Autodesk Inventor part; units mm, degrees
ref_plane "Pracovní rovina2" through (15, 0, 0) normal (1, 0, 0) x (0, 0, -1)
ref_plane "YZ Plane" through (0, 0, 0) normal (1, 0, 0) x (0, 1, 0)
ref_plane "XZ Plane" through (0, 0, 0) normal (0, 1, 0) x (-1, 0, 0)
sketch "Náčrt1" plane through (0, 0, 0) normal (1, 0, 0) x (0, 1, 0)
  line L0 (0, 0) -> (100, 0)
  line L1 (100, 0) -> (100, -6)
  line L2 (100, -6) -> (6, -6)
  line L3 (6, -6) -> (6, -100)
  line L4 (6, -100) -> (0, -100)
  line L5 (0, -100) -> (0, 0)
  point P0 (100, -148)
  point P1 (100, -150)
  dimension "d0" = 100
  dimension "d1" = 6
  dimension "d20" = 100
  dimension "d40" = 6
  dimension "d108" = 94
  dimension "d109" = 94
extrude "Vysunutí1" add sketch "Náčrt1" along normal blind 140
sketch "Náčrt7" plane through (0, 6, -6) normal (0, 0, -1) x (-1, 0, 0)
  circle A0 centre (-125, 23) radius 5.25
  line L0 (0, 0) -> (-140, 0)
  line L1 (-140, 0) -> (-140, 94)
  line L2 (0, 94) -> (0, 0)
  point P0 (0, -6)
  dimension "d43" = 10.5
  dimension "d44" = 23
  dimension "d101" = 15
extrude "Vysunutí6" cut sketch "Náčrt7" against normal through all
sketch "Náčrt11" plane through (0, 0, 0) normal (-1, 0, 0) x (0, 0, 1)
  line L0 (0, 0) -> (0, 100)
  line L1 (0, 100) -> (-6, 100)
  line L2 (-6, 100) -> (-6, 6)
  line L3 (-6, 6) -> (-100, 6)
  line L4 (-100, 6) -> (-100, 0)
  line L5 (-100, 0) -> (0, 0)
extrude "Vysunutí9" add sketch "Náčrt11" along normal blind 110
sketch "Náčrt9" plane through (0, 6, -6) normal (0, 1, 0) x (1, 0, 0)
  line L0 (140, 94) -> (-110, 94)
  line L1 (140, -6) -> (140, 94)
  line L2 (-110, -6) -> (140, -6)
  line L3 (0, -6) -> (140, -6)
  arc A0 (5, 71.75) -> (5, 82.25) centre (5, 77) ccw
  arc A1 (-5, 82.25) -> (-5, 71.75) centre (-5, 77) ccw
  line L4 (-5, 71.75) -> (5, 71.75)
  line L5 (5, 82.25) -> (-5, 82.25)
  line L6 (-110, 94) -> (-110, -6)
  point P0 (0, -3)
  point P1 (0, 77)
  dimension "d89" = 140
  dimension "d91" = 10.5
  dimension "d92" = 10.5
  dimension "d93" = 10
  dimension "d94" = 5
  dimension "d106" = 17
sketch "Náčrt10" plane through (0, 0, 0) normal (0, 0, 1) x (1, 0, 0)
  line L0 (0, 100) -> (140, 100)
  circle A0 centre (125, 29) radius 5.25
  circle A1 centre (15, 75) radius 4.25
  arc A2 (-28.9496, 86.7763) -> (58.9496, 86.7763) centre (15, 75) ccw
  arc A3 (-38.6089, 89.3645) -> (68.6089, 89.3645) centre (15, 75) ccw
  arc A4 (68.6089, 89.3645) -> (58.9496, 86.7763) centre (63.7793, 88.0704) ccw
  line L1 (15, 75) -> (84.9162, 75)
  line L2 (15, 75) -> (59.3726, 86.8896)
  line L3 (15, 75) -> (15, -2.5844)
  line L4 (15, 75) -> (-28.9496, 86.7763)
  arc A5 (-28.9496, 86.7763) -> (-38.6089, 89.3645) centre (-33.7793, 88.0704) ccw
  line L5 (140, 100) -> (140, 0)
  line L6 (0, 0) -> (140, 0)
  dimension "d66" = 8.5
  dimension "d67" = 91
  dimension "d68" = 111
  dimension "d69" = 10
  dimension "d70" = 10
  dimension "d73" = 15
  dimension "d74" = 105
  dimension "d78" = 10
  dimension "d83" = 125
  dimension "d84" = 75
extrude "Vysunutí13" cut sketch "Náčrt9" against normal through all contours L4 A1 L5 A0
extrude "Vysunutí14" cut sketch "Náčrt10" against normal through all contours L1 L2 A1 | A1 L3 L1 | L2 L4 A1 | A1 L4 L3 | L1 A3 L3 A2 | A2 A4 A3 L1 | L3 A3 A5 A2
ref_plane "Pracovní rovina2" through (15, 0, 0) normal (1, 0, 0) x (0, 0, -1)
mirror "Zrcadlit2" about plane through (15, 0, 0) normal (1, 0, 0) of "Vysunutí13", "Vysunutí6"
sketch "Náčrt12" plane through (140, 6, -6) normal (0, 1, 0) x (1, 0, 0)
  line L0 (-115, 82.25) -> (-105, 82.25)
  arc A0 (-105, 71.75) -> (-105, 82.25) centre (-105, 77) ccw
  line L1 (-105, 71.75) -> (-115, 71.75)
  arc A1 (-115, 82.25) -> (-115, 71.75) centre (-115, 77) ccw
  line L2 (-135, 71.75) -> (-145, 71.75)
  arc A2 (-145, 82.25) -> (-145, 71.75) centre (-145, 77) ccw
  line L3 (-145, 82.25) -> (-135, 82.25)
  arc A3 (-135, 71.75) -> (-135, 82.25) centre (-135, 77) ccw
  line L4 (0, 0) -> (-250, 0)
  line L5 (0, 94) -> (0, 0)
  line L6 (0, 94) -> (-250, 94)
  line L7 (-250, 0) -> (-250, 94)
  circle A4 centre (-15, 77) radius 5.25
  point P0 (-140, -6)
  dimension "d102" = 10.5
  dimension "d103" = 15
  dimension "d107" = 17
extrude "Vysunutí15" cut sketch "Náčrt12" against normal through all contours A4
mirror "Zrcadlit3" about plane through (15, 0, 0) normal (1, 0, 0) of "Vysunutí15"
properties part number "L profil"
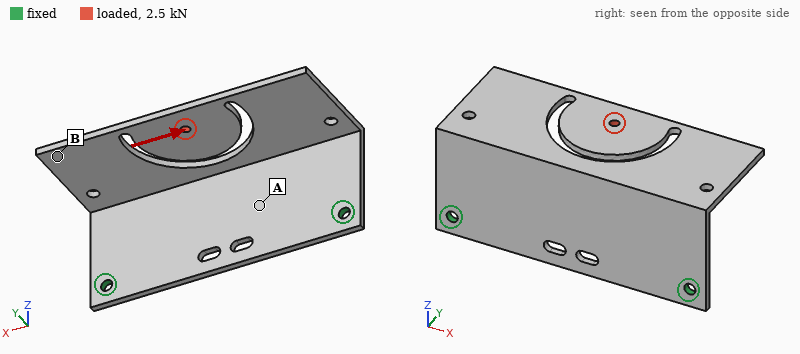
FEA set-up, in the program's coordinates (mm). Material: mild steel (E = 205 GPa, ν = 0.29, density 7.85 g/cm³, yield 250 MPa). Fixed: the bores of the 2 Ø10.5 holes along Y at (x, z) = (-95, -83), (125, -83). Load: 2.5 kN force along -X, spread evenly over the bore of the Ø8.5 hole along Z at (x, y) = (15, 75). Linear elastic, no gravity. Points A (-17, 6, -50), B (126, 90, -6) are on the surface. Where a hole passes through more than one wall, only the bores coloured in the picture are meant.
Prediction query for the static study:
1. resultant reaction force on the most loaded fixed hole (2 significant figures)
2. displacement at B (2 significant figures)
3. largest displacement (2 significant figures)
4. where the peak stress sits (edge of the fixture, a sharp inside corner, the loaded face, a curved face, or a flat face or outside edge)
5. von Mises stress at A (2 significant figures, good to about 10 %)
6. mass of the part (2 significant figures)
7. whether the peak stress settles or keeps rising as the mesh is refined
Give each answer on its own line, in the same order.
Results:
1.7 kN
0.51 mm
0.58 mm
edge of the fixture
31 MPa
2.2 kg
keeps rising
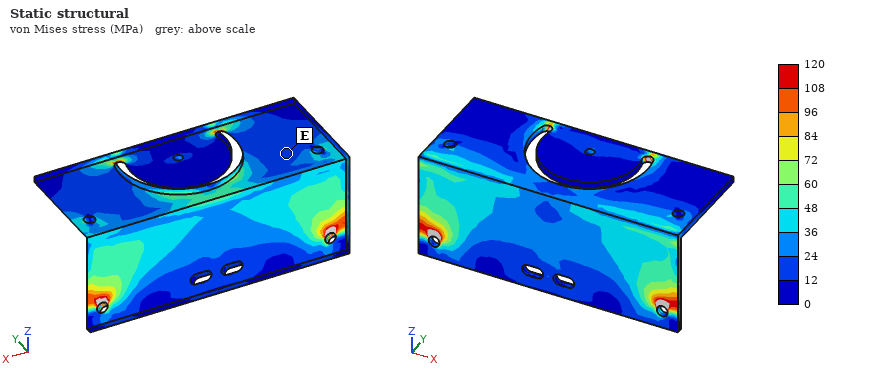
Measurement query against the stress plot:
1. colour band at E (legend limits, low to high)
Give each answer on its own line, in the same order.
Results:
12 to 24 MPa
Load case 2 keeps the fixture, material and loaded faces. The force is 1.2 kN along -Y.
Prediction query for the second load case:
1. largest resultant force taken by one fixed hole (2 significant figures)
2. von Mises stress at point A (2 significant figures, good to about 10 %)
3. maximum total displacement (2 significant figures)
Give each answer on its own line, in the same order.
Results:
600 N
18 MPa
0.81 mm
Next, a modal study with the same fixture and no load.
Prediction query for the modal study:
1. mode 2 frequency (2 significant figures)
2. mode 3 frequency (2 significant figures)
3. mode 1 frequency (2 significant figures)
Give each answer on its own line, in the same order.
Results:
330 Hz
390 Hz
170 Hz
